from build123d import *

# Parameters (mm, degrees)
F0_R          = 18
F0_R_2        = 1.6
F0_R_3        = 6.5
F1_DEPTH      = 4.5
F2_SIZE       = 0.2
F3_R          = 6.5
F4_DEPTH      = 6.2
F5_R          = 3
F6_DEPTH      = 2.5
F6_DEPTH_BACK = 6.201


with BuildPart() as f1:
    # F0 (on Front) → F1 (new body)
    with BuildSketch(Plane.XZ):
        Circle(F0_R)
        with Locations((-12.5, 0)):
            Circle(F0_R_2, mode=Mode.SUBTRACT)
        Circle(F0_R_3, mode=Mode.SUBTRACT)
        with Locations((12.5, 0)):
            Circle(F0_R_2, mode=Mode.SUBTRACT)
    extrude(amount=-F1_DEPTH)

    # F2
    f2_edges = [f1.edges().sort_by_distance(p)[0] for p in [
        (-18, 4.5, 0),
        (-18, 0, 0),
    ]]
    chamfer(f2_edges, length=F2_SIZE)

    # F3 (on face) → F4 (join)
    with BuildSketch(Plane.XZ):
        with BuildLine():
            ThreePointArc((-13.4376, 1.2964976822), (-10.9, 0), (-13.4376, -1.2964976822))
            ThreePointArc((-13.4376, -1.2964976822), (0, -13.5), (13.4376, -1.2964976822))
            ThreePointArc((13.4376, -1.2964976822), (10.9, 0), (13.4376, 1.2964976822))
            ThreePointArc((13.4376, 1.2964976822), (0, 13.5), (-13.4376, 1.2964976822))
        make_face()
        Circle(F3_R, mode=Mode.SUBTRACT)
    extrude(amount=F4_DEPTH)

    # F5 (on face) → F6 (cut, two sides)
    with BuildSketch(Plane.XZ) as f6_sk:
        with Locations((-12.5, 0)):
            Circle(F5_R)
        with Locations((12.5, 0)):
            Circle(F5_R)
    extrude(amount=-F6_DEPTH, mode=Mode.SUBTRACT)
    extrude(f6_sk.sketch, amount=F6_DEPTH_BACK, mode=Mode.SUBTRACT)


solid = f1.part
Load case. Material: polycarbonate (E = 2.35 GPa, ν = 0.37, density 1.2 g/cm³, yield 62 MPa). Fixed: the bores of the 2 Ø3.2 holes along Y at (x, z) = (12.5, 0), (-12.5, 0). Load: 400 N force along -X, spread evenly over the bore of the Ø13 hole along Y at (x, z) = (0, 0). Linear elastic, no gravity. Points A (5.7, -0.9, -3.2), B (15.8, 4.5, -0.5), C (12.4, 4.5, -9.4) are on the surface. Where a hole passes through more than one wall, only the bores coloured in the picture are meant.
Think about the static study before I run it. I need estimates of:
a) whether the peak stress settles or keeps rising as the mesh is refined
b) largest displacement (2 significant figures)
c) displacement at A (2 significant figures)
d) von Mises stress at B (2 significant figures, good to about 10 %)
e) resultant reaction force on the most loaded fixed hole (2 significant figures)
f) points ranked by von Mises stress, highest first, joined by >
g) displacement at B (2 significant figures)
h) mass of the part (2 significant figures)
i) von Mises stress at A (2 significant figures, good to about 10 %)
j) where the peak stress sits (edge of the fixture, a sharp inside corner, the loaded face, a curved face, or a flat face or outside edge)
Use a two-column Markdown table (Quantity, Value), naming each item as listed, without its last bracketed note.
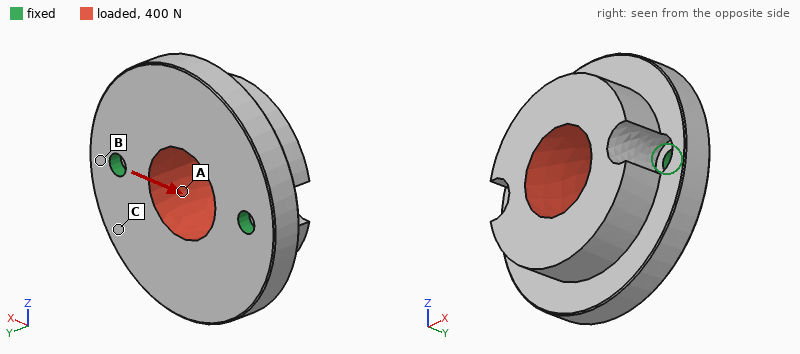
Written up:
| Quantity | Value |
|---|---|
| whether the peak stress settles or keeps rising as the mesh is refined | keeps rising |
| largest displacement | 44 µm |
| displacement at A | 30 µm |
| von Mises stress at B | 5.7 MPa |
| resultant reaction force on the most loaded fixed hole | 210 N |
| points ranked by von Mises stress, highest first, joined by > | B > A > C |
| displacement at B | 9.7 µm |
| mass of the part | 7.5 g |
| von Mises stress at A | 3.2 MPa |
| where the peak stress sits | edge of the fixture |
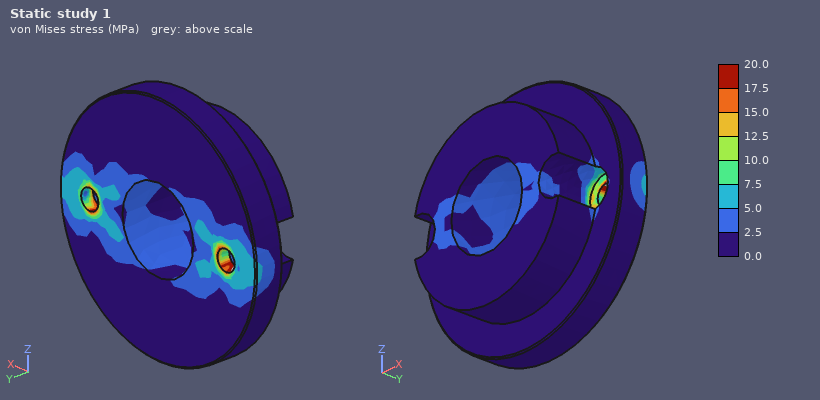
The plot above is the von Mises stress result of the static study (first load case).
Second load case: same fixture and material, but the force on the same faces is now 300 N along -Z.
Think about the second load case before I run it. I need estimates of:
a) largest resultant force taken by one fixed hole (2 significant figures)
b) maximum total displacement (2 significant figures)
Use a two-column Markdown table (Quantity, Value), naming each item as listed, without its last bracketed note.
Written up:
| Quantity | Value |
|---|---|
| largest resultant force taken by one fixed hole | 150 N |
| maximum total displacement | 0.43 mm |
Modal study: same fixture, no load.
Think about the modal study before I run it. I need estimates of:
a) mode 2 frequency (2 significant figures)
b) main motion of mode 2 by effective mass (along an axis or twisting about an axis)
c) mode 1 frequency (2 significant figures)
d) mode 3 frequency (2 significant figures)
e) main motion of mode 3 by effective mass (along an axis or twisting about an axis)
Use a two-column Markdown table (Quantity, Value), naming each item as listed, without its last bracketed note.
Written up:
| Quantity | Value |
|---|---|
| mode 2 frequency | 4600 Hz |
| main motion of mode 2 by effective mass | along Y |
| mode 1 frequency | 1400 Hz |
| mode 3 frequency | 6200 Hz |
| main motion of mode 3 by effective mass | twisting about Y |
